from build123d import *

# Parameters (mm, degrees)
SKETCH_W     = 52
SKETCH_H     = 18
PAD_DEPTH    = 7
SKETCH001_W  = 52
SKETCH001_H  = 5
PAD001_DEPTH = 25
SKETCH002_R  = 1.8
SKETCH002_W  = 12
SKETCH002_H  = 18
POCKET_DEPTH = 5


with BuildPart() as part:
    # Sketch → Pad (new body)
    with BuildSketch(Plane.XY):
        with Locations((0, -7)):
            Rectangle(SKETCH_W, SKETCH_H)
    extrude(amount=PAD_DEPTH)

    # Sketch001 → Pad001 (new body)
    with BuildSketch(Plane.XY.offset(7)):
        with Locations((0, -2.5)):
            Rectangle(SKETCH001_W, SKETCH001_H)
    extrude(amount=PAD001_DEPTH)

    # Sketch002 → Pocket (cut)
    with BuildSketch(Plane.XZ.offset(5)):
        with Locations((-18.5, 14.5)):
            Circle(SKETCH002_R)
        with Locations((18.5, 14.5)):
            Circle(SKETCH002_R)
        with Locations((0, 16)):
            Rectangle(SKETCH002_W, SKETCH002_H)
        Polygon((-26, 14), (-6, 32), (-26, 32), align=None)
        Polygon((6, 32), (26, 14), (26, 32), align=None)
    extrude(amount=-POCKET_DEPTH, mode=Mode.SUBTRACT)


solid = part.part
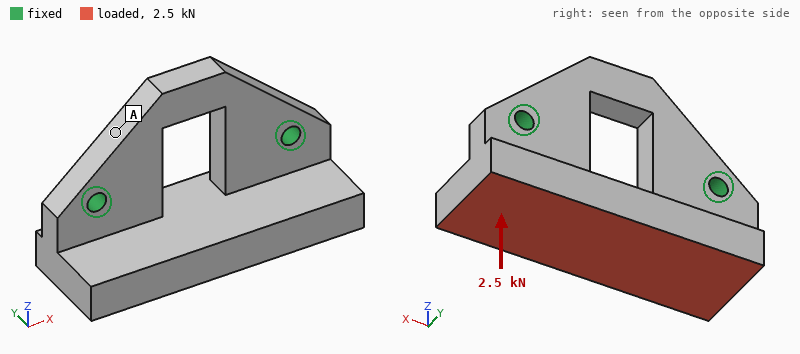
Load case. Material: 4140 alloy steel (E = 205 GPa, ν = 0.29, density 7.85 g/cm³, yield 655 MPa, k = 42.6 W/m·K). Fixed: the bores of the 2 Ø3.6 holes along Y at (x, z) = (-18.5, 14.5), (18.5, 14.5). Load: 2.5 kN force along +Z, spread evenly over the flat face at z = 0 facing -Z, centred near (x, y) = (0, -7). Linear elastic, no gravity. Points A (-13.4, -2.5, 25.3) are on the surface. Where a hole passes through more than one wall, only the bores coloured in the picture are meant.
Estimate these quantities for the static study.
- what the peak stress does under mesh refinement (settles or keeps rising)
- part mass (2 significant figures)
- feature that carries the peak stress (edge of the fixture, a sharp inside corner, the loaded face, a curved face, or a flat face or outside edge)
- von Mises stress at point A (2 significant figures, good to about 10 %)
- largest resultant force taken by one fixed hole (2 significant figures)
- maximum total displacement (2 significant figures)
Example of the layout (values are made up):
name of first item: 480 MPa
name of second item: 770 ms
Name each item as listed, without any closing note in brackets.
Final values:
what the peak stress does under mesh refinement: keeps rising
part mass: 79 g
feature that carries the peak stress: edge of the fixture
von Mises stress at point A: 14 MPa
largest resultant force taken by one fixed hole: 1.3 kN
maximum total displacement: 27 µm
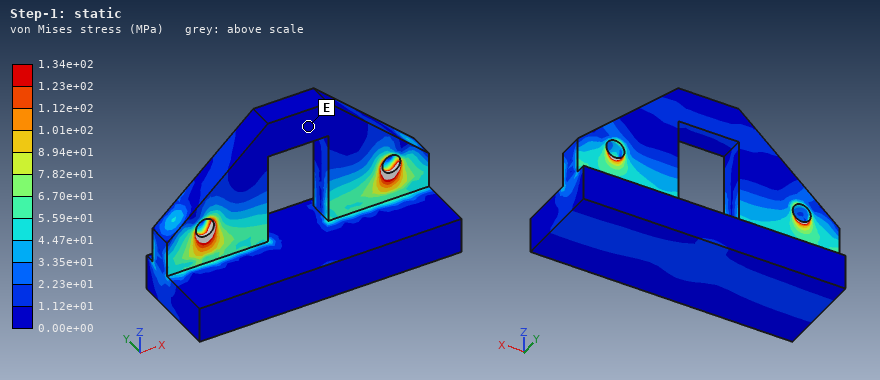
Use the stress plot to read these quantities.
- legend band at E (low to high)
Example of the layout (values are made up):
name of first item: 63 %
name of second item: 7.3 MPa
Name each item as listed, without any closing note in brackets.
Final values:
legend band at E: 0.00e+00 to 1.12e+01 MPa
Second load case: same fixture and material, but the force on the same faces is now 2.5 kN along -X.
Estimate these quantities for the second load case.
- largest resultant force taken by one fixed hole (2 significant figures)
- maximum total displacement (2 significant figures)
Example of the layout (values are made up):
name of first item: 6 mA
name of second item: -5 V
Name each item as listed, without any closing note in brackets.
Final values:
largest resultant force taken by one fixed hole: 1.5 kN
maximum total displacement: 6.5 µm
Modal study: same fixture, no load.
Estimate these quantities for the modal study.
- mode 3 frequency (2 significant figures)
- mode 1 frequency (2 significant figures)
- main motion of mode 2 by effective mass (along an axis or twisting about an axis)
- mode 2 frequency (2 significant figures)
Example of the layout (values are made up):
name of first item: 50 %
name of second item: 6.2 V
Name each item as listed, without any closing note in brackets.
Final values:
mode 3 frequency: 12 kHz
mode 1 frequency: 6000 Hz
main motion of mode 2 by effective mass: along Y
mode 2 frequency: 11 kHz
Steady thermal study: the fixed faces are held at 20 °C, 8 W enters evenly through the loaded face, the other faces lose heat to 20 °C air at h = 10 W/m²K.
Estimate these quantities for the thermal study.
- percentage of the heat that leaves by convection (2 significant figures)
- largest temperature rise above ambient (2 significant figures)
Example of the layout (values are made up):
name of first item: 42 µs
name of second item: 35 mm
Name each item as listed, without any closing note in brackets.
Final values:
percentage of the heat that leaves by convection: 3.4 %
largest temperature rise above ambient: 14 K
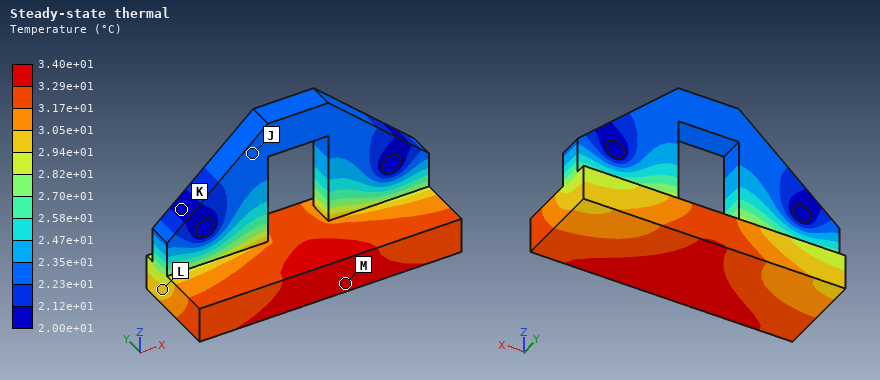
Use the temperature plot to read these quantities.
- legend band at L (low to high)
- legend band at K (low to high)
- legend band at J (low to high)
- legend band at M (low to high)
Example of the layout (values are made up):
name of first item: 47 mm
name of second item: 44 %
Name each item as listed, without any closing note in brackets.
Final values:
legend band at L: 2.94e+01 to 3.05e+01 °C
legend band at K: 2.00e+01 to 2.12e+01 °C
legend band at J: 2.23e+01 to 2.35e+01 °C
legend band at M: 3.29e+01 to 3.40e+01 °C
